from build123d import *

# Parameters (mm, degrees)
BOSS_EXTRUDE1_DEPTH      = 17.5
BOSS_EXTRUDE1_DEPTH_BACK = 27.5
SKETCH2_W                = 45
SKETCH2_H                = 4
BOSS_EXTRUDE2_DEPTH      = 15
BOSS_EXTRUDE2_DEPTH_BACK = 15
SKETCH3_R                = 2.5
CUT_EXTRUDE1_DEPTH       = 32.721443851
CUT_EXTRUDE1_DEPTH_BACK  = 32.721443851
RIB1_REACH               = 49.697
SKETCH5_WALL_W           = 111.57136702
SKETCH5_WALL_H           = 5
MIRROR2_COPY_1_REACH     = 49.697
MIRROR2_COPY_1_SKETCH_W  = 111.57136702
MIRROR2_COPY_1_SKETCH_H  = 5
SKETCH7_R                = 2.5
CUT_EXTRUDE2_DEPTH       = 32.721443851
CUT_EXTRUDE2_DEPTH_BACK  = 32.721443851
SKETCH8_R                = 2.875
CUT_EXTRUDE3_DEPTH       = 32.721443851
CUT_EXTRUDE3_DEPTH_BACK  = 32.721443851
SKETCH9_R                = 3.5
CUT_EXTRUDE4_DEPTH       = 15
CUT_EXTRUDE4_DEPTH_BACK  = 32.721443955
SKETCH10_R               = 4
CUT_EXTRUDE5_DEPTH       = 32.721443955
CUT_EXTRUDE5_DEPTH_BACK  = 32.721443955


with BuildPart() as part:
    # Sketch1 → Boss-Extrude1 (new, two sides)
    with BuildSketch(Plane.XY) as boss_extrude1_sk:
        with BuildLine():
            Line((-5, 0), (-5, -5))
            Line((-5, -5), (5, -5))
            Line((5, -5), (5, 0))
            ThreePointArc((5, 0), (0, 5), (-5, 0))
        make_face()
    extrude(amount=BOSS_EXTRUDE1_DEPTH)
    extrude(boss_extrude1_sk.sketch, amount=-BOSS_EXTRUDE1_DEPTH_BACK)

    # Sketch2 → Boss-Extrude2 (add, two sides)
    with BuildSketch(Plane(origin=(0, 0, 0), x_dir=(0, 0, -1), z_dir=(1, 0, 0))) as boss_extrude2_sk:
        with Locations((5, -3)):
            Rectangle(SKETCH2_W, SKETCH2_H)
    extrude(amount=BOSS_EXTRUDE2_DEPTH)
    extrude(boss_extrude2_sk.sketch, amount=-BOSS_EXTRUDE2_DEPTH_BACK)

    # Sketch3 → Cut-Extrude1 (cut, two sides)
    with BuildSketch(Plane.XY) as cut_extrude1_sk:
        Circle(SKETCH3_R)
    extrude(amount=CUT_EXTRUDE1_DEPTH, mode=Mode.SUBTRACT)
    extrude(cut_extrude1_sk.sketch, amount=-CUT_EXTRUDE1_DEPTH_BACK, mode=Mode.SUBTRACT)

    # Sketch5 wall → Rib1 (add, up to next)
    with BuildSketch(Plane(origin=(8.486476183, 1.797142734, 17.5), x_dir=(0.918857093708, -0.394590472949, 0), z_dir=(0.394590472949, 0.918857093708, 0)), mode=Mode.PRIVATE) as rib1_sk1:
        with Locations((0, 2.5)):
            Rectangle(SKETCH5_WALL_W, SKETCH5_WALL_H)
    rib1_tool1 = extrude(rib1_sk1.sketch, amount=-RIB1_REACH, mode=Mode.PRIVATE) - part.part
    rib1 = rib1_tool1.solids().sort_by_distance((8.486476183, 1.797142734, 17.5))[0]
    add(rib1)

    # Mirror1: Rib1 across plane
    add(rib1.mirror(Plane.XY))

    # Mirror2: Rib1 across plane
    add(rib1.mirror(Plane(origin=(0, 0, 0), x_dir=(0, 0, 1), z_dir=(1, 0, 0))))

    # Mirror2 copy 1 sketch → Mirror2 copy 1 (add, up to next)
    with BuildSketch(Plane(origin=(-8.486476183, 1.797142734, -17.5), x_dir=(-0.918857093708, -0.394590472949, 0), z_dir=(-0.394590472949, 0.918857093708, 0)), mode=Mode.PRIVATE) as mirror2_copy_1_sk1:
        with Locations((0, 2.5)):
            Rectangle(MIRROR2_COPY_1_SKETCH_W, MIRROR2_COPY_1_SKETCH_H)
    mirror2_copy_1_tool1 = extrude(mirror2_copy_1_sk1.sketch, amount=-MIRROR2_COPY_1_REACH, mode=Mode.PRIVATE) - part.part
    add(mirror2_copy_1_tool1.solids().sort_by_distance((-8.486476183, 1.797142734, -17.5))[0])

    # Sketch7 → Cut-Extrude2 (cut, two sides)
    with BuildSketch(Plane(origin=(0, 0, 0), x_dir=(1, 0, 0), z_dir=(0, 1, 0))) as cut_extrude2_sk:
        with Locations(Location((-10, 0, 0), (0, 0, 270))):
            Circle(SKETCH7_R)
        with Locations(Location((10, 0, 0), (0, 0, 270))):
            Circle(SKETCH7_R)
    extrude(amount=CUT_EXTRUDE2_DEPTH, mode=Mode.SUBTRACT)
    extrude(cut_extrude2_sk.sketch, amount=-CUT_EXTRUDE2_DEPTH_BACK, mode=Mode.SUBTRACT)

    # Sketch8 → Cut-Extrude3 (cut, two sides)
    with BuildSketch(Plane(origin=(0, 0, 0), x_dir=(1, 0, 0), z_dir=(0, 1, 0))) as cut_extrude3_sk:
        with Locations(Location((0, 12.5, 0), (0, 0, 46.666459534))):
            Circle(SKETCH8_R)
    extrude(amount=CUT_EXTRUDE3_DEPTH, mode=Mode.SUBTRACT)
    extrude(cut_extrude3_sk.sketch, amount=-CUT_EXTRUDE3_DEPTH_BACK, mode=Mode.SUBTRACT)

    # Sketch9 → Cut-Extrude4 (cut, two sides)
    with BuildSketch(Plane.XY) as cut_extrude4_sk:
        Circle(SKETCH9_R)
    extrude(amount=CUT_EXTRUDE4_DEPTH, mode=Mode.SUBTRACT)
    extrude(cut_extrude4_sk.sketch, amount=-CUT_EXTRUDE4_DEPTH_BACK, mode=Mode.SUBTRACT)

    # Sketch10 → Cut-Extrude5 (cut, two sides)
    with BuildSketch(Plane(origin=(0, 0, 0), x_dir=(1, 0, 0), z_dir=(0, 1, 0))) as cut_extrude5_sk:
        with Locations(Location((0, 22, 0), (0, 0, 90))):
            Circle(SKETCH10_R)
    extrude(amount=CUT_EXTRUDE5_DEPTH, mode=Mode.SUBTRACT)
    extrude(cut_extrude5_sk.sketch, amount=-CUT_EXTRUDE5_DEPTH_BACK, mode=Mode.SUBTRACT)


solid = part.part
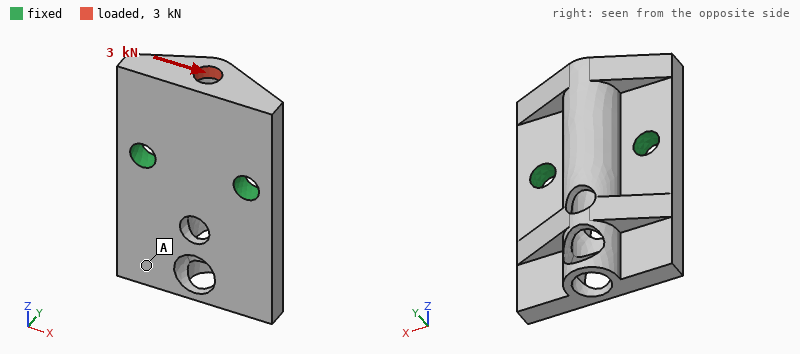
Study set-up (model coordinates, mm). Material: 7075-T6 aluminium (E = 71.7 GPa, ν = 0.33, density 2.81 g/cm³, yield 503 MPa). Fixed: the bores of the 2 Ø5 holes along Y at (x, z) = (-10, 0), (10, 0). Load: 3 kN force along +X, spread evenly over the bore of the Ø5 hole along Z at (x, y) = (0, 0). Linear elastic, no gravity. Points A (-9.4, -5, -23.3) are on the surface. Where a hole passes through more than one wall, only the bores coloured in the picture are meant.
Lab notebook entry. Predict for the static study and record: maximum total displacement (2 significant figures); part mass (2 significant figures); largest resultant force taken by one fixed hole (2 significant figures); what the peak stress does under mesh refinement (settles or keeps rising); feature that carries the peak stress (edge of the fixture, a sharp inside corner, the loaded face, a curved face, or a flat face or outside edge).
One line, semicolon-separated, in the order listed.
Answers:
39 µm; 17 g; 2.6 kN; keeps rising; edge of the fixture
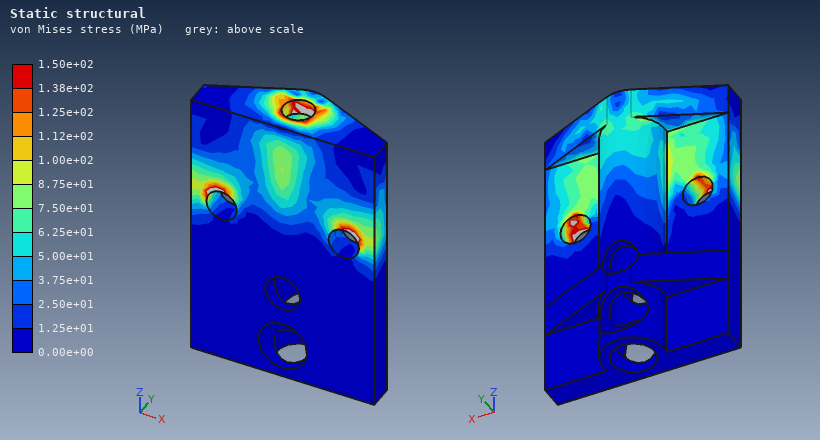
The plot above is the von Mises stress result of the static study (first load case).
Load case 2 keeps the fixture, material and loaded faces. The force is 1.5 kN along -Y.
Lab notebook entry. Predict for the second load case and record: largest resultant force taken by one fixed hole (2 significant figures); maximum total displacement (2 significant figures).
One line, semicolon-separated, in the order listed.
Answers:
790 N; 0.12 mm
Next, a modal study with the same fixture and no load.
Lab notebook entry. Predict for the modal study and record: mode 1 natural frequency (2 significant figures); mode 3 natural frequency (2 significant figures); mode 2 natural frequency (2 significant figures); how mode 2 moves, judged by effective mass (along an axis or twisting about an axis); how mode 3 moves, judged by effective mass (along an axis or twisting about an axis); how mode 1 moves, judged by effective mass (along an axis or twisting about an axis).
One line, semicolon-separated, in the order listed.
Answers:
6000 Hz; 13 kHz; 11 kHz; twisting about Z; along Y; along Y
